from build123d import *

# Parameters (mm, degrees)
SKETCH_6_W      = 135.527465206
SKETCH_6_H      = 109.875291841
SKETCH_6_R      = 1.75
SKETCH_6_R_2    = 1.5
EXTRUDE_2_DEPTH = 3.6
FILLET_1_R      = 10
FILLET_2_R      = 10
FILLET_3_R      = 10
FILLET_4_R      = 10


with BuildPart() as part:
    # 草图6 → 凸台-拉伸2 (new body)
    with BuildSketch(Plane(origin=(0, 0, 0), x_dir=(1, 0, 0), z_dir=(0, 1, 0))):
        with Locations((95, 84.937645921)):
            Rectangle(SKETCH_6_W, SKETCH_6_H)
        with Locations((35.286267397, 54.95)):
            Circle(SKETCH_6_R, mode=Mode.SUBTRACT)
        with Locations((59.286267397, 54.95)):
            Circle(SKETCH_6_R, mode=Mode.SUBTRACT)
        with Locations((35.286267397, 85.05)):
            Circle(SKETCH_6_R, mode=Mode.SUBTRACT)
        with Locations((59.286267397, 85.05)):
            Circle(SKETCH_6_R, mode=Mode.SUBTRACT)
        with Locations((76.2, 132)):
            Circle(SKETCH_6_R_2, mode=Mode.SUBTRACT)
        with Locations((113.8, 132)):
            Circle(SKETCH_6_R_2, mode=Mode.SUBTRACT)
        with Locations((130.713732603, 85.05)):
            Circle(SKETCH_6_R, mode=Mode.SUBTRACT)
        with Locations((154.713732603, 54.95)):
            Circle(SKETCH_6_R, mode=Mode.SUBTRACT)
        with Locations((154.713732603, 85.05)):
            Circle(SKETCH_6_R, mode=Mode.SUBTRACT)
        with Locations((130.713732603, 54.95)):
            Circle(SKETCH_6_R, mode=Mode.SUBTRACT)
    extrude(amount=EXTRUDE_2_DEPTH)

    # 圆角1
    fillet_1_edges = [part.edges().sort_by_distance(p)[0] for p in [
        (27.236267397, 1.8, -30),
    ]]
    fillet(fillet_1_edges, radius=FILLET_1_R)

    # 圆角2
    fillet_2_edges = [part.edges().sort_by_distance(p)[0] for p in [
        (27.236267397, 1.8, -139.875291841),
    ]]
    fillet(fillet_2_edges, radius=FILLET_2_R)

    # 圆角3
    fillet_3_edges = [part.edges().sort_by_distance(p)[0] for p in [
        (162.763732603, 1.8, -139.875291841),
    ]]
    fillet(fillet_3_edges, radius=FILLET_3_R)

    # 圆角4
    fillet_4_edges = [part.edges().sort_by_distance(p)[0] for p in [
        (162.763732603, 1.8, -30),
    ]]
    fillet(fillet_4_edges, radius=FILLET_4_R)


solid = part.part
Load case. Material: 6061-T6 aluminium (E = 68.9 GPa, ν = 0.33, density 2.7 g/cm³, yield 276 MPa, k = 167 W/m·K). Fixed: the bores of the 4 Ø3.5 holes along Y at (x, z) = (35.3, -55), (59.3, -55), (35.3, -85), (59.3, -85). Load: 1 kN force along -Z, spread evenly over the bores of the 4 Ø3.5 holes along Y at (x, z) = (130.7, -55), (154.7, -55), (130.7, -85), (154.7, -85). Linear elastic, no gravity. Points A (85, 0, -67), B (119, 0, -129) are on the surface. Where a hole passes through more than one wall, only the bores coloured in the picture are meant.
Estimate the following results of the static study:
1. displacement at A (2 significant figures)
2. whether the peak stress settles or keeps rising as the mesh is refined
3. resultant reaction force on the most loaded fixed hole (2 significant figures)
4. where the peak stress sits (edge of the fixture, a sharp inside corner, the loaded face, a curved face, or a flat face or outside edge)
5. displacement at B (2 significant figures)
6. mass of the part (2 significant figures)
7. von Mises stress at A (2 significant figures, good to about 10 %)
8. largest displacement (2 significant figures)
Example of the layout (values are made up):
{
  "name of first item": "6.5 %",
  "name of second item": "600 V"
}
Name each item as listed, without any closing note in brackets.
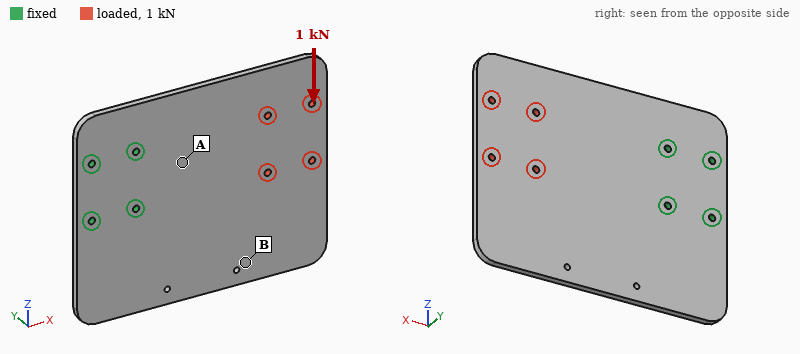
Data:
{
  "displacement at A": "13 µm",
  "whether the peak stress settles or keeps rising as the mesh is refined": "keeps rising",
  "resultant reaction force on the most loaded fixed hole": "1.7 kN",
  "where the peak stress sits": "edge of the fixture",
  "displacement at B": "40 µm",
  "mass of the part": "140 g",
  "von Mises stress at A": "11 MPa",
  "largest displacement": "59 µm"
}
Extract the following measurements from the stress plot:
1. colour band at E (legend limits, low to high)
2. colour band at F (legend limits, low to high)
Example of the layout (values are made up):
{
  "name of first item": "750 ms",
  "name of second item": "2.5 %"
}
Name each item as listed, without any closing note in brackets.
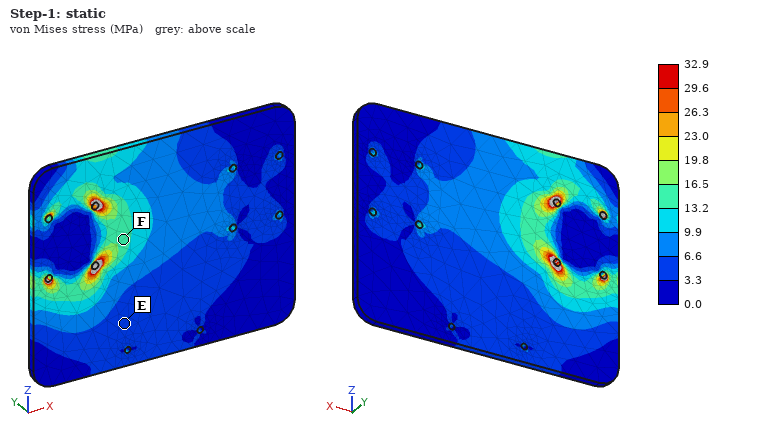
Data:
{
  "colour band at E": "3.3 to 6.6 MPa",
  "colour band at F": "13.2 to 16.5 MPa"
}
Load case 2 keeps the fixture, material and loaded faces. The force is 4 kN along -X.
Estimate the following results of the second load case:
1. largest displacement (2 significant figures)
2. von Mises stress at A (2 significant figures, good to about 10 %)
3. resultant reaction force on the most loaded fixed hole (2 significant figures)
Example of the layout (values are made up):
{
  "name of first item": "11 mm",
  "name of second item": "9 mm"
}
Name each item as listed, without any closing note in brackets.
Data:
{
  "largest displacement": "24 µm",
  "von Mises stress at A": "17 MPa",
  "resultant reaction force on the most loaded fixed hole": "1.5 kN"
}
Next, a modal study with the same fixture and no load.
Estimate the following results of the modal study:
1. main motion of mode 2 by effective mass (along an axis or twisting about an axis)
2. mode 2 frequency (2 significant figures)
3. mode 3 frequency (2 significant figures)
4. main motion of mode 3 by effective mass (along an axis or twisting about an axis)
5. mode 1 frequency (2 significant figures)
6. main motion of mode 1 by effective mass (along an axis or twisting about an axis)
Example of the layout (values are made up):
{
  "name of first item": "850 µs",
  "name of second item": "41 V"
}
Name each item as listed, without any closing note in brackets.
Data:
{
  "main motion of mode 2 by effective mass": "twisting about X",
  "mode 2 frequency": "520 Hz",
  "mode 3 frequency": "1100 Hz",
  "main motion of mode 3 by effective mass": "along Y",
  "mode 1 frequency": "260 Hz",
  "main motion of mode 1 by effective mass": "along Y"
}
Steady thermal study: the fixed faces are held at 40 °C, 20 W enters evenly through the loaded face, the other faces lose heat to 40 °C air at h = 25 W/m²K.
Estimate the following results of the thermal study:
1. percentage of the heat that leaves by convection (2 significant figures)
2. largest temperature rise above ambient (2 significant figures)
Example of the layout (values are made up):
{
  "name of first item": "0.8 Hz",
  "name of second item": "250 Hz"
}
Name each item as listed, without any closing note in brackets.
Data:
{
  "percentage of the heat that leaves by convection": "40 %",
  "largest temperature rise above ambient": "26 K"
}
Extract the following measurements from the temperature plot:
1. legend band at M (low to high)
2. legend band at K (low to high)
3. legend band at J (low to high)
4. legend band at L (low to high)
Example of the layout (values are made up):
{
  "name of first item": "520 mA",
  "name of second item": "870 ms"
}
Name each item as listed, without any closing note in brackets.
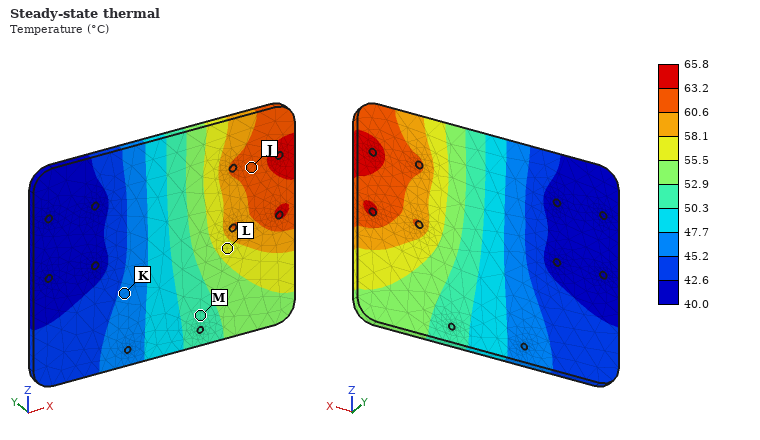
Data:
{
  "legend band at M": "50.3 to 52.9 °C",
  "legend band at K": "45.2 to 47.7 °C",
  "legend band at J": "60.6 to 63.2 °C",
  "legend band at L": "55.5 to 58.1 °C"
}
